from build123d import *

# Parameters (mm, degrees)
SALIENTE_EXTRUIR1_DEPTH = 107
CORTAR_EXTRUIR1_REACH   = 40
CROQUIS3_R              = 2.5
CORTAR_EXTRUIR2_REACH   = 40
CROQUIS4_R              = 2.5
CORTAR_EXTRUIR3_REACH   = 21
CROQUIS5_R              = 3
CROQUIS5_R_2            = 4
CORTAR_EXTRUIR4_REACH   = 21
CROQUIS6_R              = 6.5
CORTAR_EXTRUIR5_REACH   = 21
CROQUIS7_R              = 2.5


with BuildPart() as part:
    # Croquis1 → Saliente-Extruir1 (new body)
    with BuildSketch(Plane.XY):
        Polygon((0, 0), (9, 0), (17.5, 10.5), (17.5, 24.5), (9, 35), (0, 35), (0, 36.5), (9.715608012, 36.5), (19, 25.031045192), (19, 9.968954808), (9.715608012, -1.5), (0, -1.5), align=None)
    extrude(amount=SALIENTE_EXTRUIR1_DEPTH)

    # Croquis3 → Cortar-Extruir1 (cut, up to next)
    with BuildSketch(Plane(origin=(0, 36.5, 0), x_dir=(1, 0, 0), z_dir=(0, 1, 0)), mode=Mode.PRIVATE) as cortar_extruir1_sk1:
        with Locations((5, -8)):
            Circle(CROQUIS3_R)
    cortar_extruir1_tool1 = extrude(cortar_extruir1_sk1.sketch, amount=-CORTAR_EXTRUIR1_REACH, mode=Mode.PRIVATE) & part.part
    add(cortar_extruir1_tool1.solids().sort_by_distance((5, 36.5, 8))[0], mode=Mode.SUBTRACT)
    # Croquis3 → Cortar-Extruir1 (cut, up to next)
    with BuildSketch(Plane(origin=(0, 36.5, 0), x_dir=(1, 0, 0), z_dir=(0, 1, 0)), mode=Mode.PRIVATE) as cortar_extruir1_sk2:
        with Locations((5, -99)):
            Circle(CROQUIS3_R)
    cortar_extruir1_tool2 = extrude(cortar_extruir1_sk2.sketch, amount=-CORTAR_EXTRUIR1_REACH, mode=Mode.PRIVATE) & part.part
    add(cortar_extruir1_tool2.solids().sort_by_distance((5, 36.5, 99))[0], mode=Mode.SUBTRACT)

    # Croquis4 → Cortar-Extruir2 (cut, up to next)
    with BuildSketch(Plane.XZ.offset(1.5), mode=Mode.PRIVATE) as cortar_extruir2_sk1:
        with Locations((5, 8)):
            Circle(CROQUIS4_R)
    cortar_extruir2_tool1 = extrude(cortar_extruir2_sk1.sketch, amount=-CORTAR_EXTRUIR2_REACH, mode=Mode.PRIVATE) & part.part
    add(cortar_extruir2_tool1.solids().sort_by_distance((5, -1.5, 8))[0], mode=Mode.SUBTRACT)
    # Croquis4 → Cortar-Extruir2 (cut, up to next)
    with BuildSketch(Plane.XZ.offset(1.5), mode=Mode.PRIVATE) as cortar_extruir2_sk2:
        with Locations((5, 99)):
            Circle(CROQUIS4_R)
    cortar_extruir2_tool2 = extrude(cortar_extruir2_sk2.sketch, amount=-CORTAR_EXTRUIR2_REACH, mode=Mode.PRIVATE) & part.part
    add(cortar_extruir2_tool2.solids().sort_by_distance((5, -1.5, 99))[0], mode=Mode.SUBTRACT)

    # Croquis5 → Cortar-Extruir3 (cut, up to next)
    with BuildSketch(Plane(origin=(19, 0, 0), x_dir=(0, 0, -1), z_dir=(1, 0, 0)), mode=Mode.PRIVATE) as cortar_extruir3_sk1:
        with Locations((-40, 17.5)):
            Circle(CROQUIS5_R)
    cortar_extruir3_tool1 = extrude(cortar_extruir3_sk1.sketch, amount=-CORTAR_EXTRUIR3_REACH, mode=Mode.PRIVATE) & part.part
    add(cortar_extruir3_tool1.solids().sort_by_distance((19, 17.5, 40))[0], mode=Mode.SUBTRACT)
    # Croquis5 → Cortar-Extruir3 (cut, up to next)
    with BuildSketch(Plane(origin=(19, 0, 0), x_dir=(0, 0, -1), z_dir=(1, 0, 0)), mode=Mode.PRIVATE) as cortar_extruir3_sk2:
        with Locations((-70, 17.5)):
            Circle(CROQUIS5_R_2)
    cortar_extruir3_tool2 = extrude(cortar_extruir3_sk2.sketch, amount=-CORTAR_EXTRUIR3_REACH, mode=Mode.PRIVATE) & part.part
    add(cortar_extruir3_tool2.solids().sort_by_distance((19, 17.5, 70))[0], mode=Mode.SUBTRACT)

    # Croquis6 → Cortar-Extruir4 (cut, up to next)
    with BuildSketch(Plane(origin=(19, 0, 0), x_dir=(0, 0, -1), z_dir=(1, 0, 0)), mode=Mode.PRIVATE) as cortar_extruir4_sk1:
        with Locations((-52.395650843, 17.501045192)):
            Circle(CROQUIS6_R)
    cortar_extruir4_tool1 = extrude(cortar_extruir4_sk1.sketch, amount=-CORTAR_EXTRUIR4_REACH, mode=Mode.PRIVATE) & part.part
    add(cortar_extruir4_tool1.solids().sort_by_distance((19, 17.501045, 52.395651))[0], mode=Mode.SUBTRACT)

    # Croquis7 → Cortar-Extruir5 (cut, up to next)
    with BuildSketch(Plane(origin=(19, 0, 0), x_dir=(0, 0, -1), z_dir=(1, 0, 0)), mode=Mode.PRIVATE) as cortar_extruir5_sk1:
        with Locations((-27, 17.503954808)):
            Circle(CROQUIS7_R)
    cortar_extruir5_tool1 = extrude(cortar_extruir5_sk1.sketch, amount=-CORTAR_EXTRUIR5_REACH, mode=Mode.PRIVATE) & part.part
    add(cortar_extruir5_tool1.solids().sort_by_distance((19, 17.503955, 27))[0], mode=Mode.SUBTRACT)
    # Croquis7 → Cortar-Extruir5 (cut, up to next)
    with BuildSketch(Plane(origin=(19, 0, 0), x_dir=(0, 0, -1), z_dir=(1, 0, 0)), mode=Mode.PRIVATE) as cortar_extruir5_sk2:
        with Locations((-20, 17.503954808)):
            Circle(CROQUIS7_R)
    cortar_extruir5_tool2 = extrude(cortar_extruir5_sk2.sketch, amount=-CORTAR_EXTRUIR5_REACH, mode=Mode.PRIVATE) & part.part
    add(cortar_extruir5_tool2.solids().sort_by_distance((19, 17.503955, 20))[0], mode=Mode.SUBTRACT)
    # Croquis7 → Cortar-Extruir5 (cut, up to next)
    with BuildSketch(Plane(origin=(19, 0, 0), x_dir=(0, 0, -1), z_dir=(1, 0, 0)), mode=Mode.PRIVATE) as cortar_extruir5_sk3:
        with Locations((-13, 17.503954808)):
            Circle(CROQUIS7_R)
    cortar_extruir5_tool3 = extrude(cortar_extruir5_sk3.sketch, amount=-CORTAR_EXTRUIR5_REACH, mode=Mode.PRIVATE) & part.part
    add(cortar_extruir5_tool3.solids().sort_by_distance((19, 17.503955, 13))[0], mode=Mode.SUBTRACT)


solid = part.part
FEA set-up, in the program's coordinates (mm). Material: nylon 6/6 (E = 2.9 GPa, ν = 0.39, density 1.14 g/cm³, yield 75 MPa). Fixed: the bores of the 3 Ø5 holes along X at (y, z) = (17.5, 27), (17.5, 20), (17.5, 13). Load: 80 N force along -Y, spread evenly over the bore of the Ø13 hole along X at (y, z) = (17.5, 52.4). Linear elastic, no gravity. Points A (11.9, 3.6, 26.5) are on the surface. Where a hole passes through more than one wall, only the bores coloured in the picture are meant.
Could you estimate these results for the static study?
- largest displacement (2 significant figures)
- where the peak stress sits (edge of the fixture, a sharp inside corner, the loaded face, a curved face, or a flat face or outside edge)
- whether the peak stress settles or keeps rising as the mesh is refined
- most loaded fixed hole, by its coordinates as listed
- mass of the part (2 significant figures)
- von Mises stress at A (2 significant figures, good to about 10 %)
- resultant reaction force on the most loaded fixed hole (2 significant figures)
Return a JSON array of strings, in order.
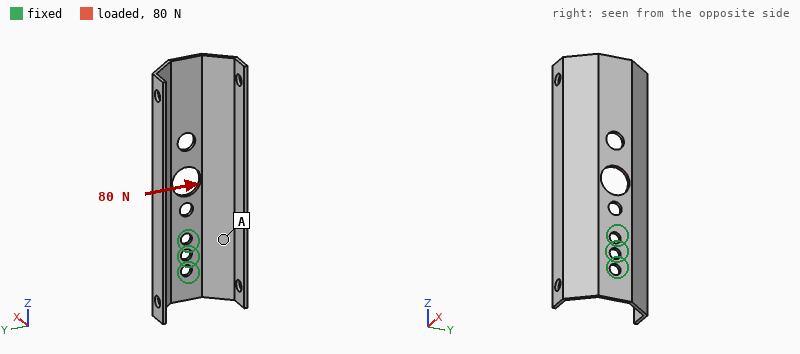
["1.2 mm", "edge of the fixture", "keeps rising", "(17.5, 27)", "11 g", "1.7 MPa", "170 N"]
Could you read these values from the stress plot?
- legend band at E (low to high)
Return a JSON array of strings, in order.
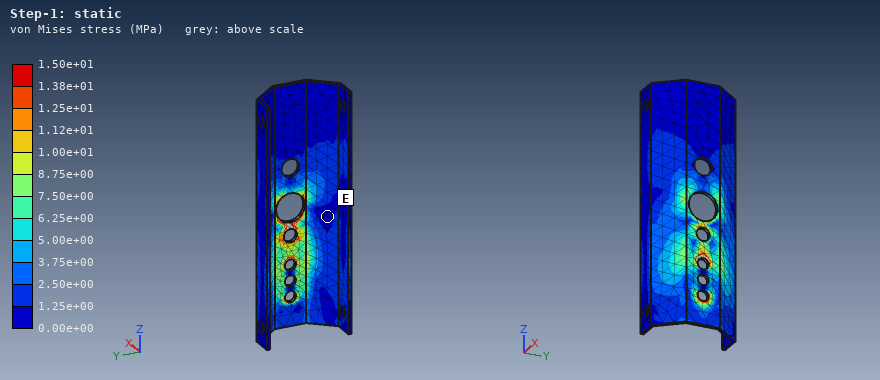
["0.00e+00 to 1.25e+00 MPa"]
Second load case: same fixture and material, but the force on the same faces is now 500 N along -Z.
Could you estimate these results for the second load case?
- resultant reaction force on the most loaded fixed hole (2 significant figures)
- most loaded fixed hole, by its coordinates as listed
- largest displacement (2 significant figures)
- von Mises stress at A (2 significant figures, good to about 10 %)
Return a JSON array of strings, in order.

["330 N", "(17.5, 27)", "1.3 mm", "3.9 MPa"]
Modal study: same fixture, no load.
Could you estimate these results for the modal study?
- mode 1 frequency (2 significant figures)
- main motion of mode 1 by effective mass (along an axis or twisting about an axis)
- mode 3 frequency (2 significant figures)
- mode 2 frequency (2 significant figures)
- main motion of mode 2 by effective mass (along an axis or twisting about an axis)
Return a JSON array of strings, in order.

["170 Hz", "along Y", "530 Hz", "230 Hz", "along X"]
